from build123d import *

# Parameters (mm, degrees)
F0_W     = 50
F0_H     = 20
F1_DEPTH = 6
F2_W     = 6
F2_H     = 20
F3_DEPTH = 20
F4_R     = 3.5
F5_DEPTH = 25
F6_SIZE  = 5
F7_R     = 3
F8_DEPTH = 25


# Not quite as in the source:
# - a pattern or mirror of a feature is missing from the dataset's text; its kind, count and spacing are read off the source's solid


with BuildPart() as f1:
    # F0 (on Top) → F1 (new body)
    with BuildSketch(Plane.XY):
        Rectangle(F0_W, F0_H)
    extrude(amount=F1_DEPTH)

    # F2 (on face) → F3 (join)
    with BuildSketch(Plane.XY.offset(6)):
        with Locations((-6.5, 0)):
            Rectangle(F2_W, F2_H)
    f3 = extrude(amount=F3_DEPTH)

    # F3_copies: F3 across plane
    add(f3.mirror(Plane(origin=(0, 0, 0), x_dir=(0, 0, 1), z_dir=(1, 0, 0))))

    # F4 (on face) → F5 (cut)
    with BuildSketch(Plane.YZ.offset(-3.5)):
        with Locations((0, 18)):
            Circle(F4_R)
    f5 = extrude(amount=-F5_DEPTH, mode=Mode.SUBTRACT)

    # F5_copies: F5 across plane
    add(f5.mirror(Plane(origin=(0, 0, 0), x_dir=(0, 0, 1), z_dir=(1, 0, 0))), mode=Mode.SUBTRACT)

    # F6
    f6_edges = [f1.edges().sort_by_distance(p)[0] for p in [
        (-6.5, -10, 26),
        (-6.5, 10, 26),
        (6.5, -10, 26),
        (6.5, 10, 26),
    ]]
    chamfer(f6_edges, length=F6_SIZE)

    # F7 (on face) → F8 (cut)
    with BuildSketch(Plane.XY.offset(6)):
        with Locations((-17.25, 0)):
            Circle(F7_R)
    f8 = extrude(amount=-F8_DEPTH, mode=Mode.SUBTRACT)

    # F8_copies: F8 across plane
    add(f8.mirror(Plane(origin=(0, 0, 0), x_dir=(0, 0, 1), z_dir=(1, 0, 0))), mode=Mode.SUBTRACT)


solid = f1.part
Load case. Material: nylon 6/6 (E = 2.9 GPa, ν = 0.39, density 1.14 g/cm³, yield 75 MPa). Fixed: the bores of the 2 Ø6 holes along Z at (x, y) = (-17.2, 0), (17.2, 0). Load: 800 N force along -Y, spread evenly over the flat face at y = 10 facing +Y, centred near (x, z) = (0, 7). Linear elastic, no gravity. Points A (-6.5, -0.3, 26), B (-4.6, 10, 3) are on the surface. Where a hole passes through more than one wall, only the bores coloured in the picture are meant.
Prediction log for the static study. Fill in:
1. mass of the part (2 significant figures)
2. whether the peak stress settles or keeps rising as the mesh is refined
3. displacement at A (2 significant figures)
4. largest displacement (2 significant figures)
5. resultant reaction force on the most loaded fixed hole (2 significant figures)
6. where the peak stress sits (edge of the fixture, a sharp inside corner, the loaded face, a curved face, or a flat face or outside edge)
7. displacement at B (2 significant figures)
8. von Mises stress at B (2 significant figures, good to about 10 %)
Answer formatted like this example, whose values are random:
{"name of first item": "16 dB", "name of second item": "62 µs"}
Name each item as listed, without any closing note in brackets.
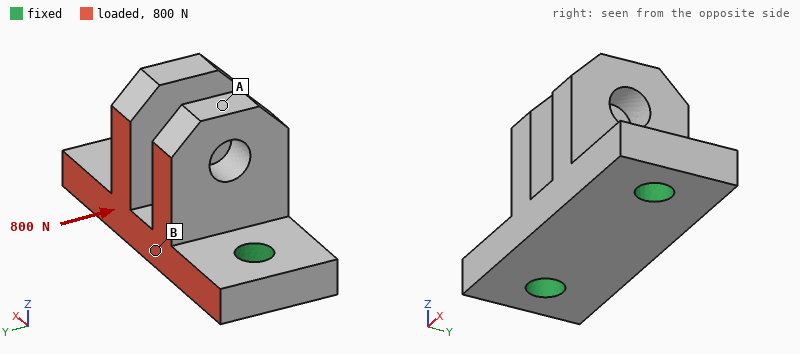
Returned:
{"mass of the part": "11 g", "whether the peak stress settles or keeps rising as the mesh is refined": "keeps rising", "displacement at A": "0.24 mm", "largest displacement": "0.24 mm", "resultant reaction force on the most loaded fixed hole": "400 N", "where the peak stress sits": "edge of the fixture", "displacement at B": "0.089 mm", "von Mises stress at B": "4.5 MPa"}
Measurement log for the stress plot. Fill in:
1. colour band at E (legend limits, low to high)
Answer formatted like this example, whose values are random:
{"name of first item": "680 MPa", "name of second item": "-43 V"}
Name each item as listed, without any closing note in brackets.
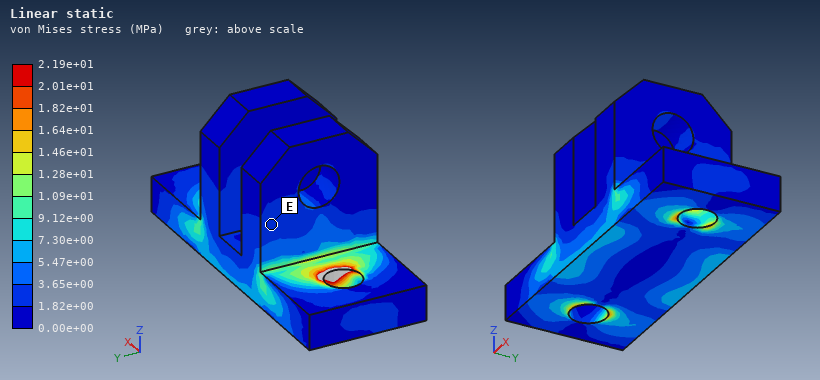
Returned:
{"colour band at E": "1.82e+00 to 3.65e+00 MPa"}
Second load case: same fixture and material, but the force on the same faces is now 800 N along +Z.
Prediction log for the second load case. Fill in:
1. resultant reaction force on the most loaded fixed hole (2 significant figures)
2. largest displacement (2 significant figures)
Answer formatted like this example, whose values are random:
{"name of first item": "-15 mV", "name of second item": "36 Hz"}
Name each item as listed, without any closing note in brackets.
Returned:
{"resultant reaction force on the most loaded fixed hole": "400 N", "largest displacement": "0.42 mm"}
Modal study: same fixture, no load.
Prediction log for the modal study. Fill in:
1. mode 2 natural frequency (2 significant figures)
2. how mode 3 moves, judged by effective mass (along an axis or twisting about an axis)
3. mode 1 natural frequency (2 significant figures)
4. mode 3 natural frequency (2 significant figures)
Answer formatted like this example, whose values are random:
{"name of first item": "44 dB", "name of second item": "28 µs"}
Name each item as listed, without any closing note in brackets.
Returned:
{"mode 2 natural frequency": "2800 Hz", "how mode 3 moves, judged by effective mass": "along X", "mode 1 natural frequency": "2800 Hz", "mode 3 natural frequency": "3400 Hz"}
